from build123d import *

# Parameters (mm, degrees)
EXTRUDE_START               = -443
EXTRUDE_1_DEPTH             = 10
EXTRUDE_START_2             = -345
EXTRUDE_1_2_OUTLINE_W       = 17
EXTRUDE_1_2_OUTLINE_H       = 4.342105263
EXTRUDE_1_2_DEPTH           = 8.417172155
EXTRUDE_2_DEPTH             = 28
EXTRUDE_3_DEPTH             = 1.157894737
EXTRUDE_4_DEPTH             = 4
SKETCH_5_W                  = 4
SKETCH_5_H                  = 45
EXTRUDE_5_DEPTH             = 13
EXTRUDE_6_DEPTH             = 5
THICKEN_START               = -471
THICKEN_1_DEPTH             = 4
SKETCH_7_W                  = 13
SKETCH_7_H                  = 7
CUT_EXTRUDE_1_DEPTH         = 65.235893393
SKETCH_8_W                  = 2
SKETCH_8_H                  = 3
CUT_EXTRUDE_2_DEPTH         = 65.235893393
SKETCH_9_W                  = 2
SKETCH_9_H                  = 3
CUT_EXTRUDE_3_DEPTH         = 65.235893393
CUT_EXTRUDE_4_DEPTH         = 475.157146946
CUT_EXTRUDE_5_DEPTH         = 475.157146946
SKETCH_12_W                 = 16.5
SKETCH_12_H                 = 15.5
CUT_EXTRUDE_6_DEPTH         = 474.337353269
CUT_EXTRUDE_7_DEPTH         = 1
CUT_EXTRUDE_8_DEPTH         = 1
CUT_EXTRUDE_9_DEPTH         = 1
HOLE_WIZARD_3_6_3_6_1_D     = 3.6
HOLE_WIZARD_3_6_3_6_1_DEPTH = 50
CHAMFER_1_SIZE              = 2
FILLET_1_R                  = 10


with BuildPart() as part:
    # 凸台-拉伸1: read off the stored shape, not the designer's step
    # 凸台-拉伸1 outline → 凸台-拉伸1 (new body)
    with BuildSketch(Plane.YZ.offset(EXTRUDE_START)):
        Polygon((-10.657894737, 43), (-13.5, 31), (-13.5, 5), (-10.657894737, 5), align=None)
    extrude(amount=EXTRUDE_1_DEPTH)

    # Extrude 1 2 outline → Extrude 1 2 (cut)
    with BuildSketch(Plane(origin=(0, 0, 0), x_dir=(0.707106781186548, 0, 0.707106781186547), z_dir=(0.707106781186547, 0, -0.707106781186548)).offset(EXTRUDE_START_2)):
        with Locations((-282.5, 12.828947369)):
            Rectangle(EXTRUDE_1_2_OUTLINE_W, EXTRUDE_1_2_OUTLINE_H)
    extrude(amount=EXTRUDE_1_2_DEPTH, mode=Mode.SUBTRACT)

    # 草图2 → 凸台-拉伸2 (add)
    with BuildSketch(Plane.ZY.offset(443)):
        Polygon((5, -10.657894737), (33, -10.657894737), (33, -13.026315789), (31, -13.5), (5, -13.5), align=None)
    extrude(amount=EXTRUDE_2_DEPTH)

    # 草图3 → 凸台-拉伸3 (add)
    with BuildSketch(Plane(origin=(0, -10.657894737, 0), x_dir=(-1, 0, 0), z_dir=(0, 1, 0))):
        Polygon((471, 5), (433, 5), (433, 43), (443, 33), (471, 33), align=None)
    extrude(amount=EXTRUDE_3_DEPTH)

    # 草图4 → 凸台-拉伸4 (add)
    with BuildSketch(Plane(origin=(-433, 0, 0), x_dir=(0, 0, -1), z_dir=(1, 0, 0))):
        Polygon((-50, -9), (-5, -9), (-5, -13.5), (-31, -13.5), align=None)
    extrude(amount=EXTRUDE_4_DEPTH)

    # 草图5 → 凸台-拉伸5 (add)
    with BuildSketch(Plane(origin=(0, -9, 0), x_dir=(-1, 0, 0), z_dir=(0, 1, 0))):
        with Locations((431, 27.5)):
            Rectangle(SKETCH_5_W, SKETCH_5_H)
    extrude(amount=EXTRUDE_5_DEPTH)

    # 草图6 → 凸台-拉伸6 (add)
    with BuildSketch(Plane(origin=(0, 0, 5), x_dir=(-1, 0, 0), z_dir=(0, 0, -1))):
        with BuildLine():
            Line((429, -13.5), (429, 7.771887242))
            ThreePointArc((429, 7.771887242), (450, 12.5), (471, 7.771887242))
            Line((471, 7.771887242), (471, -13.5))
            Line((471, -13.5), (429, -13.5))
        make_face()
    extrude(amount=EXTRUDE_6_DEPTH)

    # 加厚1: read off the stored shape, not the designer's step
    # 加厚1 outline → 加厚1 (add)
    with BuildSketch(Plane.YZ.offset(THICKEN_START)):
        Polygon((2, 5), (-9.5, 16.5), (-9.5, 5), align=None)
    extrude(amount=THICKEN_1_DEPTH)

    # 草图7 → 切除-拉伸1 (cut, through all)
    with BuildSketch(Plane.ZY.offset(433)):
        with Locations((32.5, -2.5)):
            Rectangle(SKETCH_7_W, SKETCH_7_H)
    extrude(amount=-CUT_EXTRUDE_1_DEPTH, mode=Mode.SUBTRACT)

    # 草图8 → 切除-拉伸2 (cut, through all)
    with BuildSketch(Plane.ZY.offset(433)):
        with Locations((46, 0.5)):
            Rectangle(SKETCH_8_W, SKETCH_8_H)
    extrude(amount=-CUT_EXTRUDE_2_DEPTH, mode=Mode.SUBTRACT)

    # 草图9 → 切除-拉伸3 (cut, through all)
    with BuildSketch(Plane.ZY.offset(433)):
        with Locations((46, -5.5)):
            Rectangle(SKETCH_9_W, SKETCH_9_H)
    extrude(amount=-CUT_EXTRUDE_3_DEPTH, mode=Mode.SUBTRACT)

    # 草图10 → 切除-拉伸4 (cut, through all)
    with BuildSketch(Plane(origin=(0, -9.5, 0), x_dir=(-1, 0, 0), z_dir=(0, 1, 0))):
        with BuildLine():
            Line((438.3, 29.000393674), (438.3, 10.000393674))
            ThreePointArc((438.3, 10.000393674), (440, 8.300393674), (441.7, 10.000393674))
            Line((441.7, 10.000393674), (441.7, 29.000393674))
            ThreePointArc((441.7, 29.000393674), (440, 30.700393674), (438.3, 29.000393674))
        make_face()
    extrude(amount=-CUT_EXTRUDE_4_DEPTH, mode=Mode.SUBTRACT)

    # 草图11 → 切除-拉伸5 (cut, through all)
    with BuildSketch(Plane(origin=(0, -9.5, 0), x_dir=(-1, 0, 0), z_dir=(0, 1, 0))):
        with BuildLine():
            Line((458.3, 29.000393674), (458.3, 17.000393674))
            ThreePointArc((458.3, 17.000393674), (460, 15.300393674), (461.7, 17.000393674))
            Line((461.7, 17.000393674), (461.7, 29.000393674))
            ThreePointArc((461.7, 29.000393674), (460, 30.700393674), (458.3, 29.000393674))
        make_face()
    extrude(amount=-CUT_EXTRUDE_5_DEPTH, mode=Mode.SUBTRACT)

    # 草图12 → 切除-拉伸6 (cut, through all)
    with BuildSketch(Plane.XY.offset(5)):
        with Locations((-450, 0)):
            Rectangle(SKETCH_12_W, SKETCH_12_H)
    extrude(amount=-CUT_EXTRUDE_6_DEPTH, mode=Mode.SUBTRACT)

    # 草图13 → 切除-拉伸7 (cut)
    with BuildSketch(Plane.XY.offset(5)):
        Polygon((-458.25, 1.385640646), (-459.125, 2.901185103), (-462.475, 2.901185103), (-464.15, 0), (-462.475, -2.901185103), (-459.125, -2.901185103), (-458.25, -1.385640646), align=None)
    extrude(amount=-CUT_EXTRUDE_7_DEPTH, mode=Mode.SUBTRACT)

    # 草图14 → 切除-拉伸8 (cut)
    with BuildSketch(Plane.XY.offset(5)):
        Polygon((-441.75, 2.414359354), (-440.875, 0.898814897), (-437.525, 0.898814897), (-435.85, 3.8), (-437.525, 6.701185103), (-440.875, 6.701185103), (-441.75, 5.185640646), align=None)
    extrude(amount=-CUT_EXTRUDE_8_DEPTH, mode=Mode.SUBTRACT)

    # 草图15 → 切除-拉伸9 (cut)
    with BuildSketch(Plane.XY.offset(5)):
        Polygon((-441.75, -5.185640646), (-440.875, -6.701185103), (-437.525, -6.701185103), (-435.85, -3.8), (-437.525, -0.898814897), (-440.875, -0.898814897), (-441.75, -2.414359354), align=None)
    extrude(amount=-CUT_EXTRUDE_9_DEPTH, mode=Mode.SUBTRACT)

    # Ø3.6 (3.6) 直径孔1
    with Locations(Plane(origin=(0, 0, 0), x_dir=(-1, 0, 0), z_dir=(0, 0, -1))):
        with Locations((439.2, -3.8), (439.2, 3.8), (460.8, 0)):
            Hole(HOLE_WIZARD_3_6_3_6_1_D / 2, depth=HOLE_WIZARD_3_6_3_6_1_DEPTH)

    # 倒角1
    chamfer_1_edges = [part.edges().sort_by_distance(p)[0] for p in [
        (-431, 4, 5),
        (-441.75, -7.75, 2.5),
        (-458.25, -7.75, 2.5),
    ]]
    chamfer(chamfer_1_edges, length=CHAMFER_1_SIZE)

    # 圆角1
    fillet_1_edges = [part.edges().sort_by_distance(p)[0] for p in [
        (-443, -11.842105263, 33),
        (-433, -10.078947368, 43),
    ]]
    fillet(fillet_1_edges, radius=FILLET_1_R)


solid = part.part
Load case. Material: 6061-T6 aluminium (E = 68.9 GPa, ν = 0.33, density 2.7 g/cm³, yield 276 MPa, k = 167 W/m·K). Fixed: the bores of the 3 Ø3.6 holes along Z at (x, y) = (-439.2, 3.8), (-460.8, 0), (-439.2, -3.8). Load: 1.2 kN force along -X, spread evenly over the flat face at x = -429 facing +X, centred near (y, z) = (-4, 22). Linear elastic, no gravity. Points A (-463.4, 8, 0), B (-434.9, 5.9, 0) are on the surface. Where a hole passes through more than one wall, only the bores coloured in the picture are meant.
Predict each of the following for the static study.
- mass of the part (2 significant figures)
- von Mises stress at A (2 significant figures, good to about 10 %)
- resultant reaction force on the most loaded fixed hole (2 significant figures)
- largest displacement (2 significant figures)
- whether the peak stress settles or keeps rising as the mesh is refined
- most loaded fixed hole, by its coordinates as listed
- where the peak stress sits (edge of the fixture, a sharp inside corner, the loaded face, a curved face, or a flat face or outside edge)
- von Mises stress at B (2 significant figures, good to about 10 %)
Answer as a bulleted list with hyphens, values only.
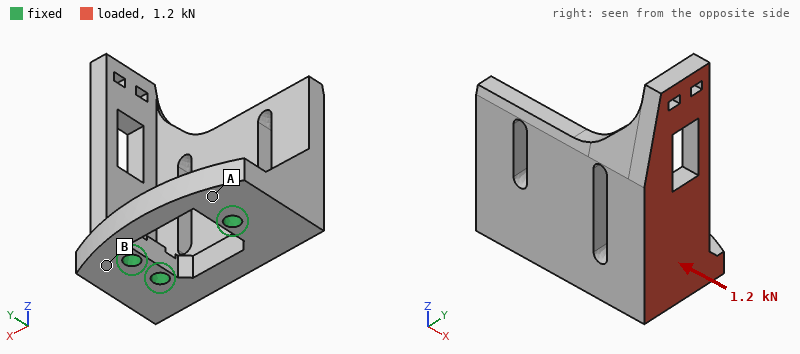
- 28 g
- 20 MPa
- 1.1 kN
- 0.36 mm
- keeps rising
- (-439.2, -3.8)
- edge of the fixture
- 43 MPa
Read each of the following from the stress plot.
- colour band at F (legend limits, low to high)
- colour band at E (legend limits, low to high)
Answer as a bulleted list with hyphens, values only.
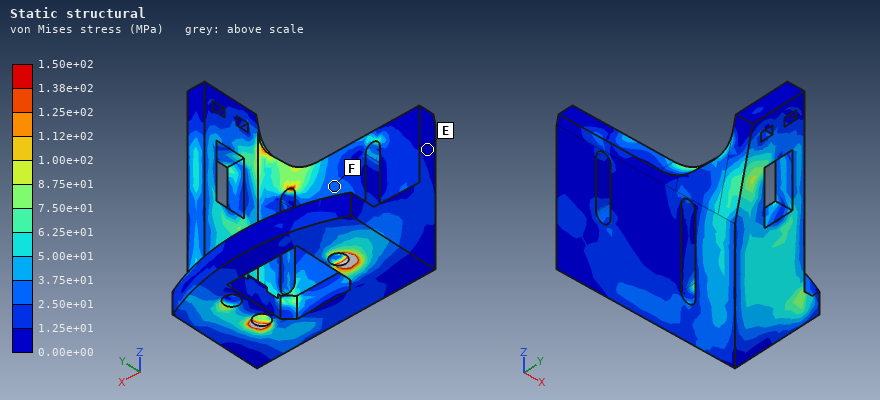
- 2.50e+01 to 3.75e+01 MPa
- 0.00e+00 to 1.25e+01 MPa
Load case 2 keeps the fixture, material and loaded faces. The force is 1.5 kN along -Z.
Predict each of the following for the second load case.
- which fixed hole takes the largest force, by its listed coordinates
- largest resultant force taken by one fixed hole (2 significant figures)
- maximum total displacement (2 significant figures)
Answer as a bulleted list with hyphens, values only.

- (-439.2, -3.8)
- 1.5 kN
- 0.12 mm
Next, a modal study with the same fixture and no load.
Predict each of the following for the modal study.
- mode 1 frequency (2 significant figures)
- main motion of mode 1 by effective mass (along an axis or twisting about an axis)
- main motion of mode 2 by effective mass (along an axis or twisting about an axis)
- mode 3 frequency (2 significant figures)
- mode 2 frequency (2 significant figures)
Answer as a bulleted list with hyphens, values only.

- 3300 Hz
- along Y
- along X
- 7000 Hz
- 3600 Hz
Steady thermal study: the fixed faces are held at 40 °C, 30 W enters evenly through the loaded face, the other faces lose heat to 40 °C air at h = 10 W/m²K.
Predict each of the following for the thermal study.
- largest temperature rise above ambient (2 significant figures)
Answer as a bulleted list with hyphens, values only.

- 45 K
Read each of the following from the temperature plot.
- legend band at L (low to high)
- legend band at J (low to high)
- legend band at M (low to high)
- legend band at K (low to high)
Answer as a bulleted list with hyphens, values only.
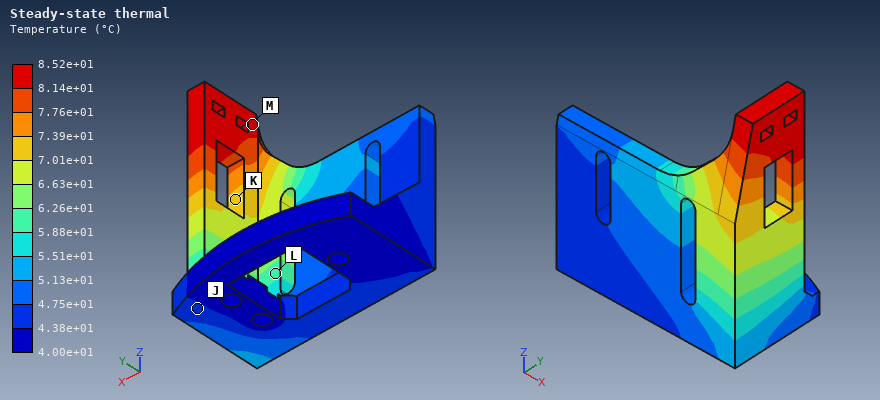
- 5.88e+01 to 6.26e+01 °C
- 4.38e+01 to 4.75e+01 °C
- 8.14e+01 to 8.52e+01 °C
- 7.01e+01 to 7.39e+01 °C
